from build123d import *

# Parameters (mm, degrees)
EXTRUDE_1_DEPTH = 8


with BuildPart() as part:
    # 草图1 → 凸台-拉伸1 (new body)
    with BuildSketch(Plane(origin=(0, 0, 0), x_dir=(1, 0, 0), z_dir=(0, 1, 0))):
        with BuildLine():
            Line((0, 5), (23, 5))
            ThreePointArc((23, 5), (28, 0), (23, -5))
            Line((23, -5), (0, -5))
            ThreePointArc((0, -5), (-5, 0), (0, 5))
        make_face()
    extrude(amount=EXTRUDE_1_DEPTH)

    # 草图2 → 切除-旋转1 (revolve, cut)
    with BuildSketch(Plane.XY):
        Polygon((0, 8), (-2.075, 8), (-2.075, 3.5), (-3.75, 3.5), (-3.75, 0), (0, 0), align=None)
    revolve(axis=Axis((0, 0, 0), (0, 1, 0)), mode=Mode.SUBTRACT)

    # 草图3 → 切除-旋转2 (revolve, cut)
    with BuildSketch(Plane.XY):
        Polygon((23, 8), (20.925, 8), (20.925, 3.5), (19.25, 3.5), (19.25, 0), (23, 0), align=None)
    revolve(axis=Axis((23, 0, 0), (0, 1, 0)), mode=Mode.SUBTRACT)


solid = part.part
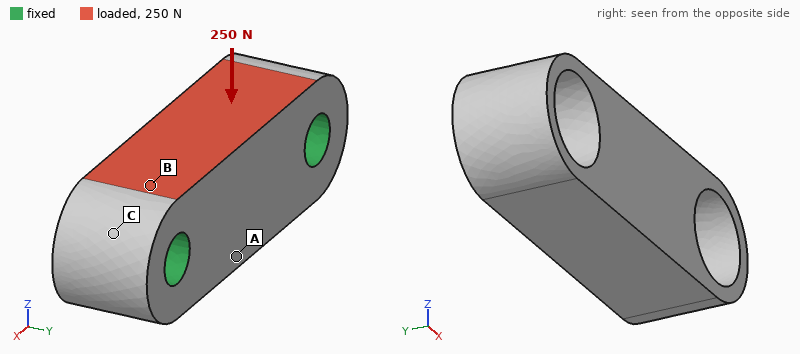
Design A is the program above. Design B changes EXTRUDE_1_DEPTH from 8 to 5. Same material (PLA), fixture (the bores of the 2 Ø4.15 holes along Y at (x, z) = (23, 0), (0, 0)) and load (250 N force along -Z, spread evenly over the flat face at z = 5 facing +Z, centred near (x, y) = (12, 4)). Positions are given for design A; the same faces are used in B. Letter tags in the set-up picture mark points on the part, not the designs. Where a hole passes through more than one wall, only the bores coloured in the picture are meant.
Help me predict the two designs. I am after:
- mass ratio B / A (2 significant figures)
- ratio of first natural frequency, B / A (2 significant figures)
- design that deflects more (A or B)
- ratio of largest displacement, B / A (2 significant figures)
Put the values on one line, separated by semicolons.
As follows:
0.59; 0.65; B; 3.3
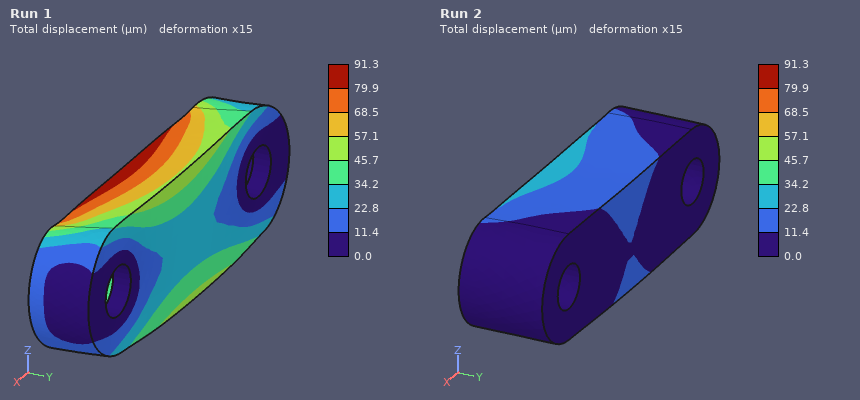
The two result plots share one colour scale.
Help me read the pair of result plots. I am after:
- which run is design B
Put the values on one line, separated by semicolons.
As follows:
Run 1
